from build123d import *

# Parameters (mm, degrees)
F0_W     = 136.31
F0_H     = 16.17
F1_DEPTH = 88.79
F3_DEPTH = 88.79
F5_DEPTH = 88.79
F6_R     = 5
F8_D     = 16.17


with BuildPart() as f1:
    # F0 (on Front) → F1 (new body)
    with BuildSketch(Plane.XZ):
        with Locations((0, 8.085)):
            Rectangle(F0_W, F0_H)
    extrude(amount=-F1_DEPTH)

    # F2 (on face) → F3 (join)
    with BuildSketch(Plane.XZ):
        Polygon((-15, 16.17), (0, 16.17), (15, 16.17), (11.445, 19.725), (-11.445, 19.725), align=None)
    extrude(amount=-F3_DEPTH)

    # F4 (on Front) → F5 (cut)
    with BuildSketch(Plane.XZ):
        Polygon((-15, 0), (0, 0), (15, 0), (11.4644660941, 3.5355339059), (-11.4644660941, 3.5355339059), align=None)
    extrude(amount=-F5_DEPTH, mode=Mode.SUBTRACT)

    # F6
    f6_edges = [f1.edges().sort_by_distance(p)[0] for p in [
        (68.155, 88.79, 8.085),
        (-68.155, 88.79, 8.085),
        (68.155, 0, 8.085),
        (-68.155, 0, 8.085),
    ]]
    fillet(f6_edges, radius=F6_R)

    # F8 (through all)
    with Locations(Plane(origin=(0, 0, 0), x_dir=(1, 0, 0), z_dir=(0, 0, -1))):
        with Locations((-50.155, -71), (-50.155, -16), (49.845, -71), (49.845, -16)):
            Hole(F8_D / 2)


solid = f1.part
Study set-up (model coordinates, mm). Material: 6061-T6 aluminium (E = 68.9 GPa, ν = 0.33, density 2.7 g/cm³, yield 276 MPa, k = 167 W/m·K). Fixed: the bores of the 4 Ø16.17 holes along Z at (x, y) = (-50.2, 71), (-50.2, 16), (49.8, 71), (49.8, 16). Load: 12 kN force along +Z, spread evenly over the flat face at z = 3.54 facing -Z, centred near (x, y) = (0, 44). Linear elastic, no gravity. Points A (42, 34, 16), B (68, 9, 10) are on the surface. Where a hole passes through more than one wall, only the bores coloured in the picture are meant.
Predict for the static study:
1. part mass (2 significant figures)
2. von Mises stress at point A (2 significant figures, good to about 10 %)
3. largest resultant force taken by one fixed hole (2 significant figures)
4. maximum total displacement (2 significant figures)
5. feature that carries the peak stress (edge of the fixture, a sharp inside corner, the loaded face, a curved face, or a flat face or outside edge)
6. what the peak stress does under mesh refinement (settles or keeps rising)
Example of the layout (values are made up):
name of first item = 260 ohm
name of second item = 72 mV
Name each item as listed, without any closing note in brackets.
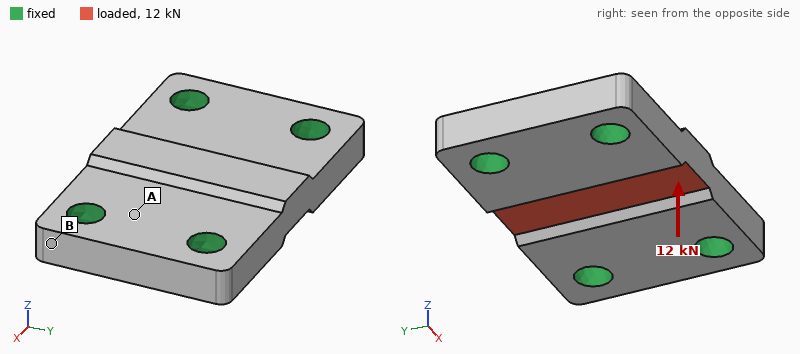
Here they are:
part mass = 490 g
von Mises stress at point A = 11 MPa
largest resultant force taken by one fixed hole = 3.5 kN
maximum total displacement = 30 µm
feature that carries the peak stress = edge of the fixture
what the peak stress does under mesh refinement = keeps rising
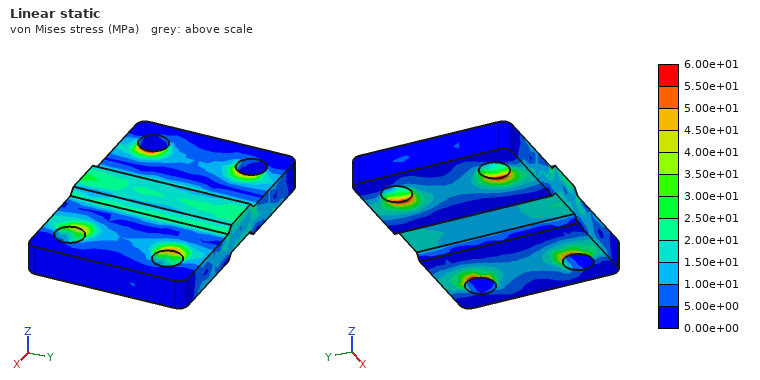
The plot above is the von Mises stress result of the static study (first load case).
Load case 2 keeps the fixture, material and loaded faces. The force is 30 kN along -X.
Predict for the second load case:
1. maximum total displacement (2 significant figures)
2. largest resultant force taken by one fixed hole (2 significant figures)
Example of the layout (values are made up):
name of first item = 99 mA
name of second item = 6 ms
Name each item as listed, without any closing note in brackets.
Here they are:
maximum total displacement = 11 µm
largest resultant force taken by one fixed hole = 7.8 kN
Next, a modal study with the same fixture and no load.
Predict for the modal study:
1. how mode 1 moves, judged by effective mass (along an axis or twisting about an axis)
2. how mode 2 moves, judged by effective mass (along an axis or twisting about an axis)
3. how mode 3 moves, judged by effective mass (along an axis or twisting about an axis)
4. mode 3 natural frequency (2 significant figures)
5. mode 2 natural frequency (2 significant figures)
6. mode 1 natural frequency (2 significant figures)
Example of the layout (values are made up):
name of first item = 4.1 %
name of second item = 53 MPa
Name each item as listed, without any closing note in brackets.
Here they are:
how mode 1 moves, judged by effective mass = along Z
how mode 2 moves, judged by effective mass = twisting about X
how mode 3 moves, judged by effective mass = along Y
mode 3 natural frequency = 15 kHz
mode 2 natural frequency = 9800 Hz
mode 1 natural frequency = 8200 Hz
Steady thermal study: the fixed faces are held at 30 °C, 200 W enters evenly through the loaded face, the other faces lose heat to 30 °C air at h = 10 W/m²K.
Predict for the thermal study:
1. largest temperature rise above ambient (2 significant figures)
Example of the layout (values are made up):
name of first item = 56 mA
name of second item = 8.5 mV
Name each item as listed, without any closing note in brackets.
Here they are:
largest temperature rise above ambient = 21 K
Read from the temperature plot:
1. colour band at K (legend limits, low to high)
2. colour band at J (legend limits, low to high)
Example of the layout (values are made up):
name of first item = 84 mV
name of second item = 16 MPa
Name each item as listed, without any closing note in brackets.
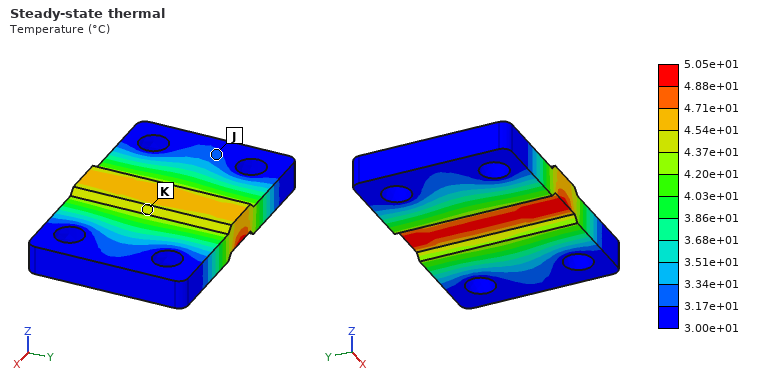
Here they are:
colour band at K = 4.37e+01 to 4.54e+01 °C
colour band at J = 3.17e+01 to 3.34e+01 °C
